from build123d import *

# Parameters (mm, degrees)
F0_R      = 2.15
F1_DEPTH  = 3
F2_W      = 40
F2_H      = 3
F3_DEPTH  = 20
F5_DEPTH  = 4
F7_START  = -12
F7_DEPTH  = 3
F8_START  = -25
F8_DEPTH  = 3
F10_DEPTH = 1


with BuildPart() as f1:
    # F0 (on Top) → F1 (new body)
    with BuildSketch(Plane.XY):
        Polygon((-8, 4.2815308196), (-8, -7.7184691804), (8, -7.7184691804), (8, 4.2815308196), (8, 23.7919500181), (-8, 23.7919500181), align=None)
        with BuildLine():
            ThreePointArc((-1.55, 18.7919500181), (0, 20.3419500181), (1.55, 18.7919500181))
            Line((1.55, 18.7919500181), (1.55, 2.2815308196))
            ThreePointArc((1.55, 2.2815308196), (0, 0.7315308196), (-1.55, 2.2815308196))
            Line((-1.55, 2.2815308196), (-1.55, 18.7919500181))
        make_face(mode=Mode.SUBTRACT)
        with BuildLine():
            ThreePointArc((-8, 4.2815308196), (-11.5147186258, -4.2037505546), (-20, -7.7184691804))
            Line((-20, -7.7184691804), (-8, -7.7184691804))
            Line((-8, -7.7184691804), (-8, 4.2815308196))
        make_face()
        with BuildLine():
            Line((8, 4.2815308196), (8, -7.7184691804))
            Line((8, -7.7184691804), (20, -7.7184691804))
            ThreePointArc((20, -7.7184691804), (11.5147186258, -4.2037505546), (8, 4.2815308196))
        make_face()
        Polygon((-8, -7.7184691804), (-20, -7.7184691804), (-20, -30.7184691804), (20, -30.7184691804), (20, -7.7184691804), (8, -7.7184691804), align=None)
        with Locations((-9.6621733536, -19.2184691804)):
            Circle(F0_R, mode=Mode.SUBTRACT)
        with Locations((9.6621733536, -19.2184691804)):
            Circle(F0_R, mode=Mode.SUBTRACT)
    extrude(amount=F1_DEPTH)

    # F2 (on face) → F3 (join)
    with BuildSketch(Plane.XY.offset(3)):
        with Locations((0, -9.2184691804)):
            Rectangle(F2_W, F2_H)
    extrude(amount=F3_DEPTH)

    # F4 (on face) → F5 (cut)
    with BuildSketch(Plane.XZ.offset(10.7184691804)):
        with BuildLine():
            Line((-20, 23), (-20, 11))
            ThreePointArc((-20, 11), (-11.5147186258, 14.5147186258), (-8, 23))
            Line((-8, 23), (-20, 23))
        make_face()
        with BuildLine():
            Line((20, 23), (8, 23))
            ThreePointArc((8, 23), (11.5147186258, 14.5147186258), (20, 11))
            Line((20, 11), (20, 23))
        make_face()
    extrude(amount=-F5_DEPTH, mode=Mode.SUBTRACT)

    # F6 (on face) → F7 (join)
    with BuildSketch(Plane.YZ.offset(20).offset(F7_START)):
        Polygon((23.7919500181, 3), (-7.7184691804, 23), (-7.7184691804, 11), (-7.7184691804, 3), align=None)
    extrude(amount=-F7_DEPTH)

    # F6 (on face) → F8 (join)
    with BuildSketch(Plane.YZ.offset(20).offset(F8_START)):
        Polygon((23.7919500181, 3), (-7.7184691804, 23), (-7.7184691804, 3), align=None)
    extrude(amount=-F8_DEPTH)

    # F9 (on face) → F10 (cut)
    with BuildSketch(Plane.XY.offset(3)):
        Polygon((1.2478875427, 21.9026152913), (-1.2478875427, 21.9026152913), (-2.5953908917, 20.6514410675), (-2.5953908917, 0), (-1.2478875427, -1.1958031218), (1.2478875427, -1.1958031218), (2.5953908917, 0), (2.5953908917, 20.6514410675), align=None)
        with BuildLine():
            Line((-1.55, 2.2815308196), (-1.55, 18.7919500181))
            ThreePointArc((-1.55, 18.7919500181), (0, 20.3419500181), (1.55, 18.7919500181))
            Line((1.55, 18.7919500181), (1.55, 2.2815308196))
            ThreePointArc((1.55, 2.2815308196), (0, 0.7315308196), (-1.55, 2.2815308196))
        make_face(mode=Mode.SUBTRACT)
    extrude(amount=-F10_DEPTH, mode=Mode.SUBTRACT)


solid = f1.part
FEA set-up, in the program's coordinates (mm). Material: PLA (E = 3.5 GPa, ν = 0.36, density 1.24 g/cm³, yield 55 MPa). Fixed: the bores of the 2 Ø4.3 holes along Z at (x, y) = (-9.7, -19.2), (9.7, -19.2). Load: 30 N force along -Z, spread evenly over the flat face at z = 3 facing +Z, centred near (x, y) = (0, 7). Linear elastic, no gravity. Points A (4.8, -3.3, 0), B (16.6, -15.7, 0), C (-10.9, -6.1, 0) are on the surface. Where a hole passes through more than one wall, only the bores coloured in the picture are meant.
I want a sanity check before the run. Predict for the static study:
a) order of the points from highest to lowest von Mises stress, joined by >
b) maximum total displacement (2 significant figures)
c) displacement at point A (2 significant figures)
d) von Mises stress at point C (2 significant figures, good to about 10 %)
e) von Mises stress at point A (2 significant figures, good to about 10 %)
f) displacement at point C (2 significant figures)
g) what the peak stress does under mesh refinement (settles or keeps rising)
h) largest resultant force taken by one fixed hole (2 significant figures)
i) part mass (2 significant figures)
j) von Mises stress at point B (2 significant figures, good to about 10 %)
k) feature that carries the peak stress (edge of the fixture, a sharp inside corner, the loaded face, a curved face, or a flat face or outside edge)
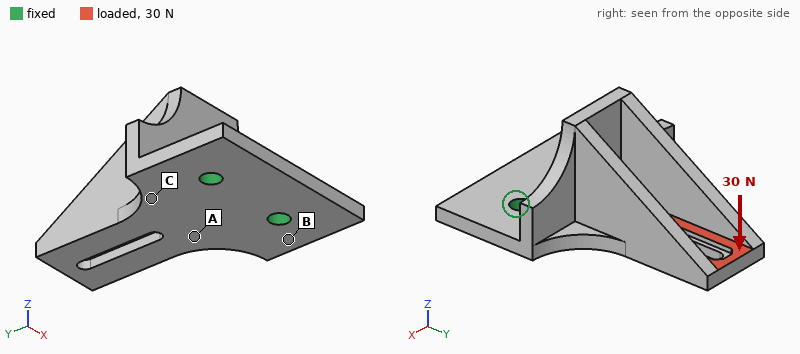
B > C > A
0.76 mm
0.21 mm
2.9 MPa
1.4 MPa
0.15 mm
keeps rising
15 N
9.6 g
7.3 MPa
edge of the fixture
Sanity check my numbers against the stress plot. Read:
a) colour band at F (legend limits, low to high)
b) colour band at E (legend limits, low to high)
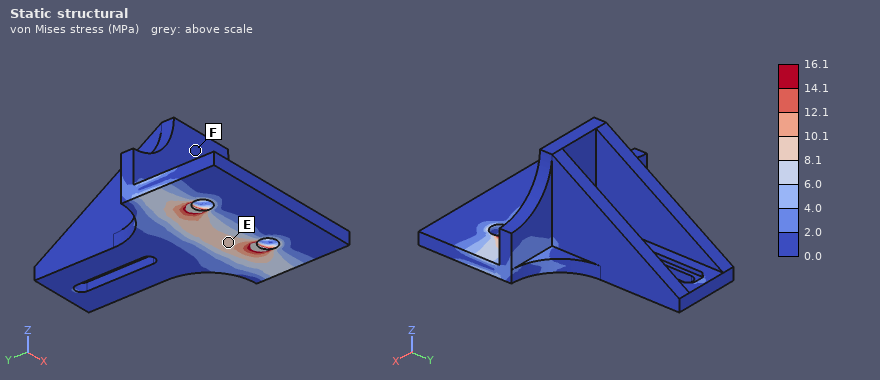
0.0 to 2.0 MPa
8.1 to 10.1 MPa
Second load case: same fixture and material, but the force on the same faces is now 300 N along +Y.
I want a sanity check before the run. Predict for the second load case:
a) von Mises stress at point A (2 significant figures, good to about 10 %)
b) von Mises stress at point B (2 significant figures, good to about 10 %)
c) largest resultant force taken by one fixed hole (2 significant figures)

2.3 MPa
4.7 MPa
160 N
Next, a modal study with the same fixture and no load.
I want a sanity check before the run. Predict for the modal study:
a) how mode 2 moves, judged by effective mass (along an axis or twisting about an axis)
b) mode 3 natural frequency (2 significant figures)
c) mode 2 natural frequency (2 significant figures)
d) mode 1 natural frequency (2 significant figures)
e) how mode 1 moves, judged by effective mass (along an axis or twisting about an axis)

along X
2700 Hz
2300 Hz
600 Hz
along Z
